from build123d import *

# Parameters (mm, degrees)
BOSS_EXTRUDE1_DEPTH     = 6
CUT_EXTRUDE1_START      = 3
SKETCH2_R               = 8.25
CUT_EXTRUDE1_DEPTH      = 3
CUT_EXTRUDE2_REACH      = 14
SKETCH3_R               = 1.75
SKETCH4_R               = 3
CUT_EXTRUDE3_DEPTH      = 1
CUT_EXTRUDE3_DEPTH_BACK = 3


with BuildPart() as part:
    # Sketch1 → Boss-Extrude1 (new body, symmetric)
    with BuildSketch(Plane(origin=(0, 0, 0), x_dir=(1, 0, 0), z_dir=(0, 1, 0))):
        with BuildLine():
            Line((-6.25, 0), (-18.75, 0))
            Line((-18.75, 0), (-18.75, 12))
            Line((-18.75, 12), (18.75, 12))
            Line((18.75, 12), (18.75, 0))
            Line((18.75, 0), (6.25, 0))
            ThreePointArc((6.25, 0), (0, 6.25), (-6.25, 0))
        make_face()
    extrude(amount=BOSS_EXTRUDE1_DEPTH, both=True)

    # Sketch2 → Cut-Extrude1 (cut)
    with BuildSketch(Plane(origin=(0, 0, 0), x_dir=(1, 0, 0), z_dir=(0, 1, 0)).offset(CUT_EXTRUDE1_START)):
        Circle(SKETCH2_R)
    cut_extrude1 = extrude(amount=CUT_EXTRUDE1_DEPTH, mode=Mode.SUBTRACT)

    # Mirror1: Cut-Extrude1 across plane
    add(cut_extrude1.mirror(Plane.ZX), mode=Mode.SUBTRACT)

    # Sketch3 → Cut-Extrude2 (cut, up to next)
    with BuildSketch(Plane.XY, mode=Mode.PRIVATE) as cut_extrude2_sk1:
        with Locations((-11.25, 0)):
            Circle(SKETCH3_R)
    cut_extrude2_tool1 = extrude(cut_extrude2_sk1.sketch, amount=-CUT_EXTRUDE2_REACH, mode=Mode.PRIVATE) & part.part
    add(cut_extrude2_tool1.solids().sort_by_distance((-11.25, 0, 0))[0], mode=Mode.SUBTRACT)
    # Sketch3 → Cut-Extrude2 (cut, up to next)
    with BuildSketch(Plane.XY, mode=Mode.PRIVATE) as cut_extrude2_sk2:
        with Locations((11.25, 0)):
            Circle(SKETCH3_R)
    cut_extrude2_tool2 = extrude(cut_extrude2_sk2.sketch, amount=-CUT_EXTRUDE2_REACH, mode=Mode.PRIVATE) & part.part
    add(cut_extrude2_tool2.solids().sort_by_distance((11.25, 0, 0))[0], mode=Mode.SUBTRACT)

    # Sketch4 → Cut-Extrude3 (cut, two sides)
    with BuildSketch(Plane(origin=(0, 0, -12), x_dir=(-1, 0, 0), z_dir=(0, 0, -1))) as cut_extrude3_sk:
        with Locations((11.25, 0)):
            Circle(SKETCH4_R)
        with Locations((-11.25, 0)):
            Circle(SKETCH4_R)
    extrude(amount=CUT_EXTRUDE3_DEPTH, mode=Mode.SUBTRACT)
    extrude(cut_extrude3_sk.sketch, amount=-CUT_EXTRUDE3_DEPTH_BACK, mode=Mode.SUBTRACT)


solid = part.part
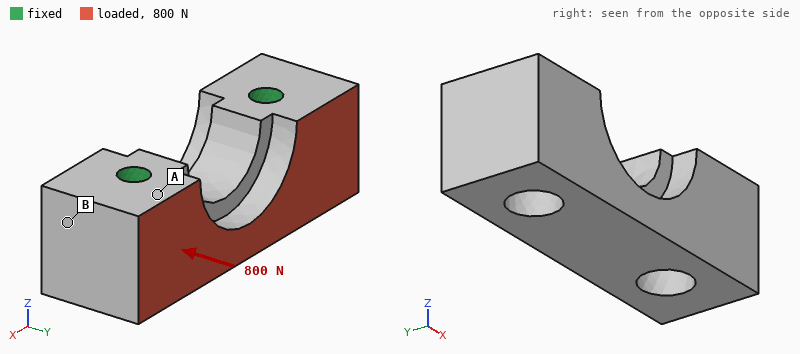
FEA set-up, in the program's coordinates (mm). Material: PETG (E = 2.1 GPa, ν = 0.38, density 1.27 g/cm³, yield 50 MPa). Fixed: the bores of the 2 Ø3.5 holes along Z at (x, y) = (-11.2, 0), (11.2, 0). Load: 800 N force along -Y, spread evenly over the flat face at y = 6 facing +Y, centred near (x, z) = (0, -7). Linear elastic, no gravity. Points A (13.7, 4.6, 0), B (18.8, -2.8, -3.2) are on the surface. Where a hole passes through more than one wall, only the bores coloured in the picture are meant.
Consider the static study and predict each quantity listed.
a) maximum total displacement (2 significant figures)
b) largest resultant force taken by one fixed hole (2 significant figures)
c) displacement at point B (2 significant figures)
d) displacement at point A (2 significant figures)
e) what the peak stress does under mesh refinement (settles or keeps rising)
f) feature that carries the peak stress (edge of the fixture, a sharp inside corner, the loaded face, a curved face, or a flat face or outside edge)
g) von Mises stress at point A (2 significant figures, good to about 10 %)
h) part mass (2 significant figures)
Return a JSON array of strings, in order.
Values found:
["42 µm", "400 N", "12 µm", "7.5 µm", "keeps rising", "edge of the fixture", "2.8 MPa", "5.1 g"]
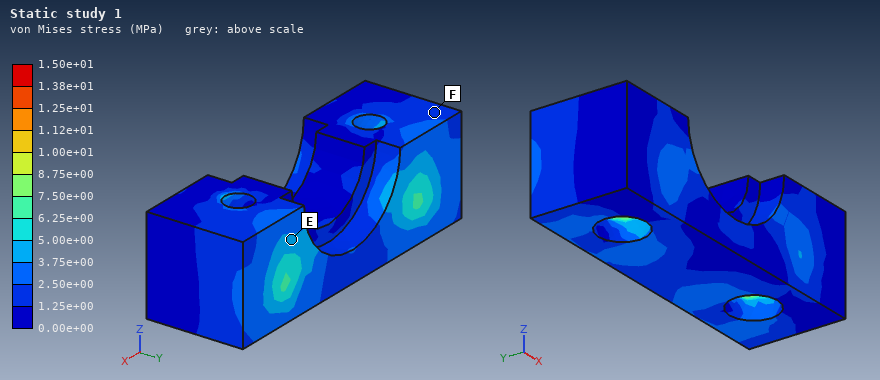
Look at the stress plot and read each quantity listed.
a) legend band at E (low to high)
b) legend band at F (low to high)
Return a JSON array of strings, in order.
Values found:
["3.75e+00 to 5.00e+00 MPa", "1.25e+00 to 2.50e+00 MPa"]
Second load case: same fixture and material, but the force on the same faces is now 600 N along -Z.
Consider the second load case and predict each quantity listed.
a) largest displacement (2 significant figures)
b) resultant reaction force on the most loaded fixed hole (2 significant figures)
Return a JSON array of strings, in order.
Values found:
["73 µm", "300 N"]
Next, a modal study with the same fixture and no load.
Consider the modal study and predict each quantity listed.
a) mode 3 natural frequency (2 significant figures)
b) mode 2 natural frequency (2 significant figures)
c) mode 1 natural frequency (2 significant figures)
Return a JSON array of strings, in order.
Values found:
["14 kHz", "13 kHz", "10 kHz"]
